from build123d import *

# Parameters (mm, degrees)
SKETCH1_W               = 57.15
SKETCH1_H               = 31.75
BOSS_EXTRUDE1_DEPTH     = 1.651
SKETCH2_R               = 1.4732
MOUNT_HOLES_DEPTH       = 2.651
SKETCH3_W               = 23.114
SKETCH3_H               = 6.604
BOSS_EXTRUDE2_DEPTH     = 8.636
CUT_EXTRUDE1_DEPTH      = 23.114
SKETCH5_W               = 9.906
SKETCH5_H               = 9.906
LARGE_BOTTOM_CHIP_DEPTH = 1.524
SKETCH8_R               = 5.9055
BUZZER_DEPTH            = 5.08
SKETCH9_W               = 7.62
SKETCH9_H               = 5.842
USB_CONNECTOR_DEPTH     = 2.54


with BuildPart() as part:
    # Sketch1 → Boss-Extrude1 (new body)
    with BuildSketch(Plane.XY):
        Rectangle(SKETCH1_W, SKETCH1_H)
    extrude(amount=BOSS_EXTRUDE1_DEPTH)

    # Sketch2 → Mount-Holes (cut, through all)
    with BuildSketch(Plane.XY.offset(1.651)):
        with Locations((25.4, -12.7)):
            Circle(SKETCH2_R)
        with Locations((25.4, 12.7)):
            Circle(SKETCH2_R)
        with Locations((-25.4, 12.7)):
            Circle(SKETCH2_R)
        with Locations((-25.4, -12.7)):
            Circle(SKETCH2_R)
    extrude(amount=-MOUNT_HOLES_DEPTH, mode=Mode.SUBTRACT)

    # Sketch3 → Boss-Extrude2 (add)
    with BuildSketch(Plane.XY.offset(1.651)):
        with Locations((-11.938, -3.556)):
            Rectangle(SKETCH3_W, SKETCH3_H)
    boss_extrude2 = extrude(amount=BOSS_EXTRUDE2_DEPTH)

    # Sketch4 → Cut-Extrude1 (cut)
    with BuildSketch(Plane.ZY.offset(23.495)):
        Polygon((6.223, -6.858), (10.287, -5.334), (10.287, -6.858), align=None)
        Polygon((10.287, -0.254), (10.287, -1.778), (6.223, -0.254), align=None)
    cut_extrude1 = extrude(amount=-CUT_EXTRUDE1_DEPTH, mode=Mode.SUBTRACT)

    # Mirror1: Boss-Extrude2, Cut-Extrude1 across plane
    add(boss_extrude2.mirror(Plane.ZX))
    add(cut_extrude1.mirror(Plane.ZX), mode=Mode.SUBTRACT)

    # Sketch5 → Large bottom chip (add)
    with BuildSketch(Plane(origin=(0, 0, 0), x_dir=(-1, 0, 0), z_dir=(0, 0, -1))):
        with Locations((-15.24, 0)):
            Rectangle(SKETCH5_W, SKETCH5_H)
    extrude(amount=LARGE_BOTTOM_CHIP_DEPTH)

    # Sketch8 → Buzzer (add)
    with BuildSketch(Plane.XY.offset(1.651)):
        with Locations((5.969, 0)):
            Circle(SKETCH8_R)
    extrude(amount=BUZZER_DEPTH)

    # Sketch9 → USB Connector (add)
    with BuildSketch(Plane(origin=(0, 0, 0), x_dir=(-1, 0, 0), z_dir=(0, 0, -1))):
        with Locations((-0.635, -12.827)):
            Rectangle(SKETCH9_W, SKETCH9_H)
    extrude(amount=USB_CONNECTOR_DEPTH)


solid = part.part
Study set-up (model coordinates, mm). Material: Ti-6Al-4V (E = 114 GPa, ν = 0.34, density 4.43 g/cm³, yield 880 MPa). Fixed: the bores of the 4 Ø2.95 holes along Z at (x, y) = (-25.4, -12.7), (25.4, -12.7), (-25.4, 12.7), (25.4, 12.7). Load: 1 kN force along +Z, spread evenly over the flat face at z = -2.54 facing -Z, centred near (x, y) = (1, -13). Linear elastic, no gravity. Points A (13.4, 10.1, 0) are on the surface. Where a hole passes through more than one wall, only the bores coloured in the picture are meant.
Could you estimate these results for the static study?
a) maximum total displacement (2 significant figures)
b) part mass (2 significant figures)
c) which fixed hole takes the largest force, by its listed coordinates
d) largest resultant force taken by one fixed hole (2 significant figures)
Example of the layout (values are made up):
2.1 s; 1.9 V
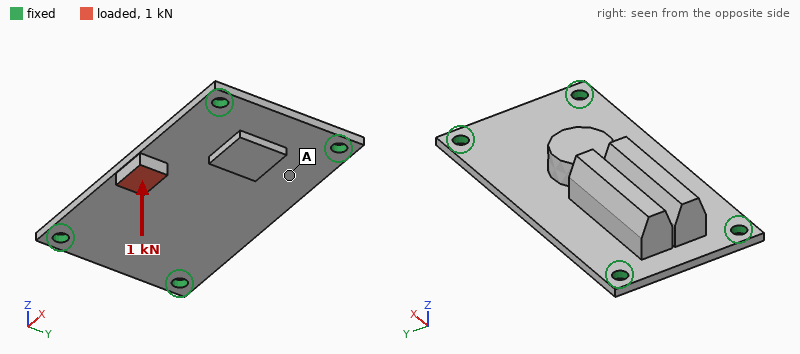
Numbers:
0.49 mm; 27 g; (-25.4, -12.7); 700 N
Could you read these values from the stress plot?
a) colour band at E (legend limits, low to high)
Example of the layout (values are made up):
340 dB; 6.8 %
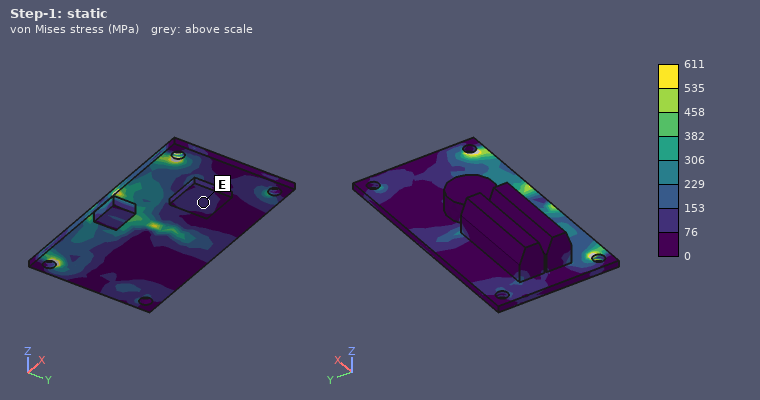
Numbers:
76 to 153 MPa
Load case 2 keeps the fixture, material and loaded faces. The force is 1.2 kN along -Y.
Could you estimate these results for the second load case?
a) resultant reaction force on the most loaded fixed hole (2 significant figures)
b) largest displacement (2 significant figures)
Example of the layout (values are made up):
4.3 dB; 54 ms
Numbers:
490 N; 0.18 mm
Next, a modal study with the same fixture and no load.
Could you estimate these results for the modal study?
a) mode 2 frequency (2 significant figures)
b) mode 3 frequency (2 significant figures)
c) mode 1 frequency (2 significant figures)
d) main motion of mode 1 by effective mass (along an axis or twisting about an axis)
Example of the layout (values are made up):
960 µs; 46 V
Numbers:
6600 Hz; 9000 Hz; 2800 Hz; along Z
